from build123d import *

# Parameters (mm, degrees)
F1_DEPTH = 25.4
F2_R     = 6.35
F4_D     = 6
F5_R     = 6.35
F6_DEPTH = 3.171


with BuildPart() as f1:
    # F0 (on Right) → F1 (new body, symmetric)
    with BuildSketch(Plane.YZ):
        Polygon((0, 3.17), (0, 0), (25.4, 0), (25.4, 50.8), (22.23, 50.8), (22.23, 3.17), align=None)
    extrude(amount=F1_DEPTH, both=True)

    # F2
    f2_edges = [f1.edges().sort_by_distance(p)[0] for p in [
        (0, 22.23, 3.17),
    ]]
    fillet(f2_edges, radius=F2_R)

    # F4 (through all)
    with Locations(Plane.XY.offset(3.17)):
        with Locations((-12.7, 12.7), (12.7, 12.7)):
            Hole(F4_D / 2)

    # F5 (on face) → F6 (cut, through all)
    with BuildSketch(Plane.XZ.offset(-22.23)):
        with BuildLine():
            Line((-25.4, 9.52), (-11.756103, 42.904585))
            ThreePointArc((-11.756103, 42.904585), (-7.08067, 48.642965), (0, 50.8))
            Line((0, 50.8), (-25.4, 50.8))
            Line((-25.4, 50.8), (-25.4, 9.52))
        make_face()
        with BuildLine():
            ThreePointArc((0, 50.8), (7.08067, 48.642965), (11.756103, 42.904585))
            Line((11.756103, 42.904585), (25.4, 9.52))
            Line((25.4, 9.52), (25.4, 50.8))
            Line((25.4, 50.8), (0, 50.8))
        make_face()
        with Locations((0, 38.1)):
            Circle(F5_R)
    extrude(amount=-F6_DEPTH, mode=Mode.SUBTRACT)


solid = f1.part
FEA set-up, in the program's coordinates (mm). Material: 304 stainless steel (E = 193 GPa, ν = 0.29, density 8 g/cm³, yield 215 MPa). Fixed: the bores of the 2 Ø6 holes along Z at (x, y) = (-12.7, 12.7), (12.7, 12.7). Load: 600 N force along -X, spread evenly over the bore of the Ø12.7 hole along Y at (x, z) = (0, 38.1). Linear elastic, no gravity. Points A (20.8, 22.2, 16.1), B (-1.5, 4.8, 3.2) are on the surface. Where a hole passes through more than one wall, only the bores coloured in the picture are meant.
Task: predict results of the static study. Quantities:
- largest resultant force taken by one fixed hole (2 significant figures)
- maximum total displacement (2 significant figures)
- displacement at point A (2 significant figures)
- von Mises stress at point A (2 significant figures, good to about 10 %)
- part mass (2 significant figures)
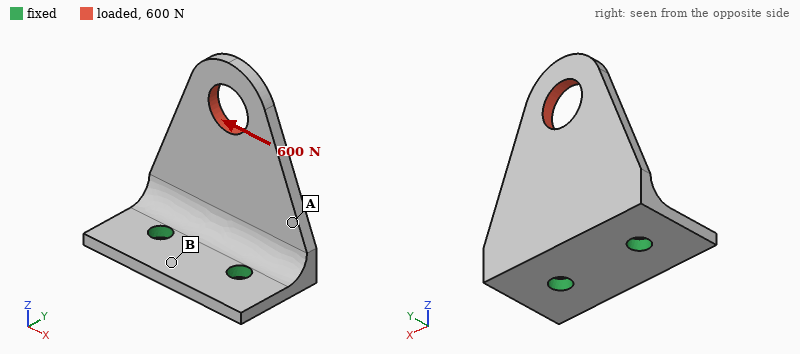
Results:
830 N
42 µm
23 µm
32 MPa
75 g
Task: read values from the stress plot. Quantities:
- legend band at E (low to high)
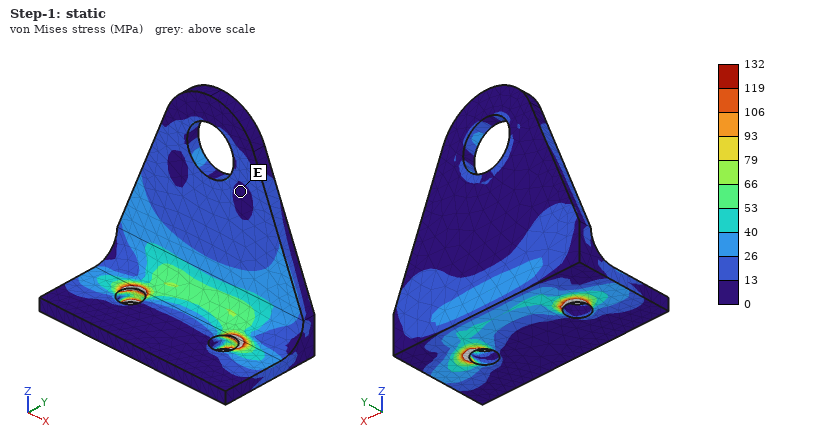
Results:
0 to 13 MPa
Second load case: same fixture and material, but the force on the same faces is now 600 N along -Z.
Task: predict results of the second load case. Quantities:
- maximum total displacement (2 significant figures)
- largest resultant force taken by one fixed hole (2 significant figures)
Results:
48 µm
300 N
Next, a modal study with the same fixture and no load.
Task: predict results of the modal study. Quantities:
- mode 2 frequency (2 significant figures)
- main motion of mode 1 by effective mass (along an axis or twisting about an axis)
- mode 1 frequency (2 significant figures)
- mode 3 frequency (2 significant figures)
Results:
4200 Hz
along Y
1500 Hz
5500 Hz
